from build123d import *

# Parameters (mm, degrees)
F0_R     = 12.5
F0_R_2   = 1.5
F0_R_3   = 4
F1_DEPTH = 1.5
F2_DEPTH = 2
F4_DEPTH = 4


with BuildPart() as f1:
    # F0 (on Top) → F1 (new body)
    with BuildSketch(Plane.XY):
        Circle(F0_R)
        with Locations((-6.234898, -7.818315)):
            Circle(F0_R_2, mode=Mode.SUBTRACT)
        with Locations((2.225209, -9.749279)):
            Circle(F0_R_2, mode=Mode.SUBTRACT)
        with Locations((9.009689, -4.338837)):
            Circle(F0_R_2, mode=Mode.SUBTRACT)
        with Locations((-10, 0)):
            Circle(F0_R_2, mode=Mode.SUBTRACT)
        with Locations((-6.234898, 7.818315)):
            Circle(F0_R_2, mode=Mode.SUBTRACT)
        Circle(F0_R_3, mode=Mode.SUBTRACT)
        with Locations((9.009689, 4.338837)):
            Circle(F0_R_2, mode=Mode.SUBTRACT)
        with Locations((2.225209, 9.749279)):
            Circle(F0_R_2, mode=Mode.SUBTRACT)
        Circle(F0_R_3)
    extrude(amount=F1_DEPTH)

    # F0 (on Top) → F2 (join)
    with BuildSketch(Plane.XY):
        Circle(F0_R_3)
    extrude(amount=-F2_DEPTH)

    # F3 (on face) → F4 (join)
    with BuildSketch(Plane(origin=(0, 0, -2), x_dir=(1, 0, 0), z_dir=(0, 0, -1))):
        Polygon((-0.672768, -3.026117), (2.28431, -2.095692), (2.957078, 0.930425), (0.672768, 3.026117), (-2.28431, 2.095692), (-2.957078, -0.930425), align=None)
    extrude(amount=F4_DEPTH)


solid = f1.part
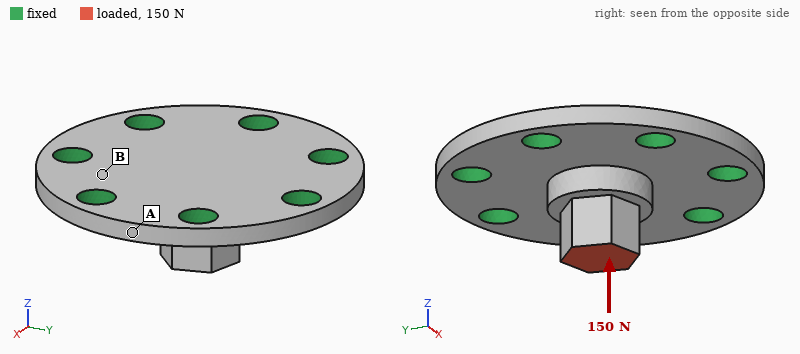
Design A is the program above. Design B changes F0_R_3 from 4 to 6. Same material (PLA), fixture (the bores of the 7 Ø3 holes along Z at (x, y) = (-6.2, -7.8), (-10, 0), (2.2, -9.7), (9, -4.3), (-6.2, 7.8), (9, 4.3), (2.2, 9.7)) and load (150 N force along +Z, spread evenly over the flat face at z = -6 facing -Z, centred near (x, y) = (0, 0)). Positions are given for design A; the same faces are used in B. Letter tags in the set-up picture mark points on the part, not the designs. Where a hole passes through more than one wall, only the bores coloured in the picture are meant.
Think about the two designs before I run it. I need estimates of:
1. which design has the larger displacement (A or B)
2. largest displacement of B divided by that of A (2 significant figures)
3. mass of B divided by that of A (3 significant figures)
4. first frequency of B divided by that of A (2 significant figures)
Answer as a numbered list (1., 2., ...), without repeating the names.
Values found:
1. A
2. 0.52
3. 1.15
4. 1.3
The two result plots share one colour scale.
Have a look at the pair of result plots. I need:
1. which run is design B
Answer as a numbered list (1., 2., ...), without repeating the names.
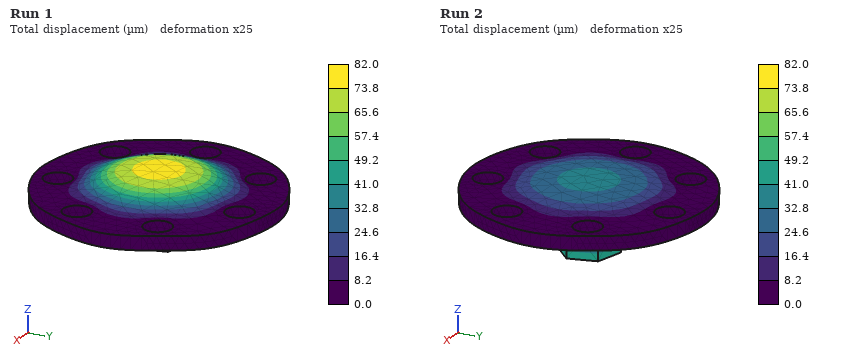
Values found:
1. Run 2
